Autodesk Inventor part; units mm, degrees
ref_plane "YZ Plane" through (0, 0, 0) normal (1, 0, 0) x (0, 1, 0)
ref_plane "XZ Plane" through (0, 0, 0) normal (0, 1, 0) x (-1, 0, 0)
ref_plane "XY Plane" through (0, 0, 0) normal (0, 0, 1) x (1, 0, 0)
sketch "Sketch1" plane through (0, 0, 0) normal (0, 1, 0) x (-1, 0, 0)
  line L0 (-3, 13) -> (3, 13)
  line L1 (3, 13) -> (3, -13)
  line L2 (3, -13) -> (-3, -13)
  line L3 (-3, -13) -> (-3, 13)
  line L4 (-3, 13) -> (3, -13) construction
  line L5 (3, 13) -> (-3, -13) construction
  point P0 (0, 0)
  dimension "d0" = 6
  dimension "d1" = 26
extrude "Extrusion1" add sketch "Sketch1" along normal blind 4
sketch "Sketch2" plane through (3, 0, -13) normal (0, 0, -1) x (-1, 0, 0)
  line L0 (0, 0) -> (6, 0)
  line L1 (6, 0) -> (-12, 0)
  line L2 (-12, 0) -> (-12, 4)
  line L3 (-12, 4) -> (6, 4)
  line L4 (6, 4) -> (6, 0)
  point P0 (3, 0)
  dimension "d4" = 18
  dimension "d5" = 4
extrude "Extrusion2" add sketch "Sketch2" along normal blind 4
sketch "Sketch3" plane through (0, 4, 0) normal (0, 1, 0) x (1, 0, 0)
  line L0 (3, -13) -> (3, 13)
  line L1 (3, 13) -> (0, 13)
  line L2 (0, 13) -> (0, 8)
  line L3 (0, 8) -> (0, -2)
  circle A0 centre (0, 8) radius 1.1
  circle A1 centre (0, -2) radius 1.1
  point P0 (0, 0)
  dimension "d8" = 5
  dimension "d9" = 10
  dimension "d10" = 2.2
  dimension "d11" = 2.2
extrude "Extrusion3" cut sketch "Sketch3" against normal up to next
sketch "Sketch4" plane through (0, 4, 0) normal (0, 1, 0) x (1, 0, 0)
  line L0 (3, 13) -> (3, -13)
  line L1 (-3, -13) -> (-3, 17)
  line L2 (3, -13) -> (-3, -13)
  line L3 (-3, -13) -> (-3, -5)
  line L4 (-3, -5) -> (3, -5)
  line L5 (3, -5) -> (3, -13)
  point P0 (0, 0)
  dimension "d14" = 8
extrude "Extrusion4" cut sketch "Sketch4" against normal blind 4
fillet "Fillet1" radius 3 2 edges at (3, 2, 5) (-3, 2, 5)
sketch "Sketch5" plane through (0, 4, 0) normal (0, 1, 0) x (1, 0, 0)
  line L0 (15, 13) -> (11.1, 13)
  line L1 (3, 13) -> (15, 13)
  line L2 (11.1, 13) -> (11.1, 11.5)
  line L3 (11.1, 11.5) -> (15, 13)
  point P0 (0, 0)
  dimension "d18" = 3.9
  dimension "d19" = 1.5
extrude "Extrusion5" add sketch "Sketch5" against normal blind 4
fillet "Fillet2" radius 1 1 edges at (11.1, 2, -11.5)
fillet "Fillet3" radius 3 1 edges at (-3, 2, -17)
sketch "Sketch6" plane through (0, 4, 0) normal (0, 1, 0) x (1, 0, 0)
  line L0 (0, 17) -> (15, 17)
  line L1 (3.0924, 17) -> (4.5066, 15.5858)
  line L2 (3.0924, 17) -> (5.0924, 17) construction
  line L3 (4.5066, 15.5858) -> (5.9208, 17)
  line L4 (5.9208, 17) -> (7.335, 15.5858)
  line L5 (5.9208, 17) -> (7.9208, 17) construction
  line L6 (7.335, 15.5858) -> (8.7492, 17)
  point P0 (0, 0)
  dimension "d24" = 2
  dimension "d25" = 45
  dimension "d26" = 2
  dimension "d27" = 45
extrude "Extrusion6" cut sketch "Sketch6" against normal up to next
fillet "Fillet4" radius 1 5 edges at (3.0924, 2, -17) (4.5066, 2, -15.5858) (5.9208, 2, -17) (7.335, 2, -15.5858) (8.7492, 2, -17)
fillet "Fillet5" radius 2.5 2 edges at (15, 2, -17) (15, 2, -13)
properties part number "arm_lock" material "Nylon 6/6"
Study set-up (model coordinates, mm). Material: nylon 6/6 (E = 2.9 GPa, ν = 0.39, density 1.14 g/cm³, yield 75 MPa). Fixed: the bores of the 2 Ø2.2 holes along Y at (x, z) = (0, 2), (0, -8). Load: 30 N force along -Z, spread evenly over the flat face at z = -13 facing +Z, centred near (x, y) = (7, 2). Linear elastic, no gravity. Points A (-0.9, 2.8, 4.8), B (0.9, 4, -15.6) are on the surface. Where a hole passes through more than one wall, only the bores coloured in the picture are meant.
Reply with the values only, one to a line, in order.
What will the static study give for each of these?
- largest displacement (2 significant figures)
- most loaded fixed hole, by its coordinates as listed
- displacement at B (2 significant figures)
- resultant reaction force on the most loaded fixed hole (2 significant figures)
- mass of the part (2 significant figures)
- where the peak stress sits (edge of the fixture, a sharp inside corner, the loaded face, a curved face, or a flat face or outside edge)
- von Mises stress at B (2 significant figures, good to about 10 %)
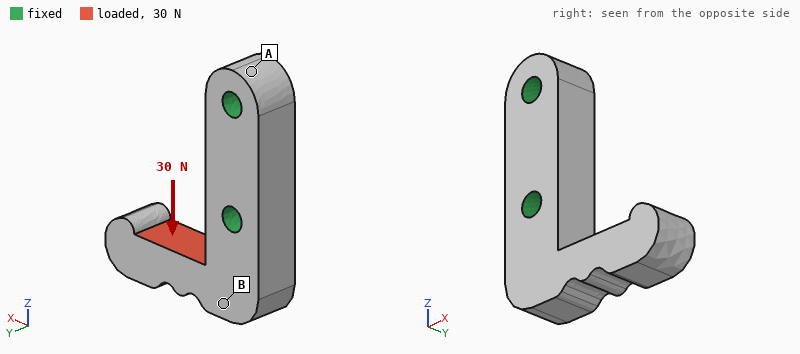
0.27 mm
(0, -8)
0.044 mm
30 N
0.73 g
a curved face
5.4 MPa
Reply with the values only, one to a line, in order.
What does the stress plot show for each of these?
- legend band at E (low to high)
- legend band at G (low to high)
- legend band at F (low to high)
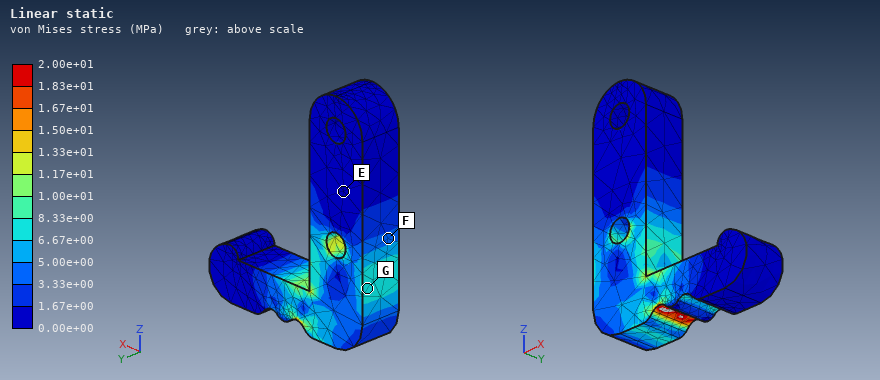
0.00e+00 to 1.67e+00 MPa
6.67e+00 to 8.33e+00 MPa
3.33e+00 to 5.00e+00 MPa
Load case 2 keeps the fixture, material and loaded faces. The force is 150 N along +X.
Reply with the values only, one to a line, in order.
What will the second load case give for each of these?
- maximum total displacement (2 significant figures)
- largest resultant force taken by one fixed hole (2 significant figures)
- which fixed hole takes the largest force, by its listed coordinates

0.20 mm
180 N
(0, -8)
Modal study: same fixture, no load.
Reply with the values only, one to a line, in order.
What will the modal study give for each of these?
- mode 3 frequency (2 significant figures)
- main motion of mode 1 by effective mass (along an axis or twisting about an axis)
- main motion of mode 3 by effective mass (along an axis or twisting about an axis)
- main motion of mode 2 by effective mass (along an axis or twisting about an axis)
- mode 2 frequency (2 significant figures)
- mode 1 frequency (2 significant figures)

9900 Hz
along Y
along X
along Z
3600 Hz
3300 Hz
